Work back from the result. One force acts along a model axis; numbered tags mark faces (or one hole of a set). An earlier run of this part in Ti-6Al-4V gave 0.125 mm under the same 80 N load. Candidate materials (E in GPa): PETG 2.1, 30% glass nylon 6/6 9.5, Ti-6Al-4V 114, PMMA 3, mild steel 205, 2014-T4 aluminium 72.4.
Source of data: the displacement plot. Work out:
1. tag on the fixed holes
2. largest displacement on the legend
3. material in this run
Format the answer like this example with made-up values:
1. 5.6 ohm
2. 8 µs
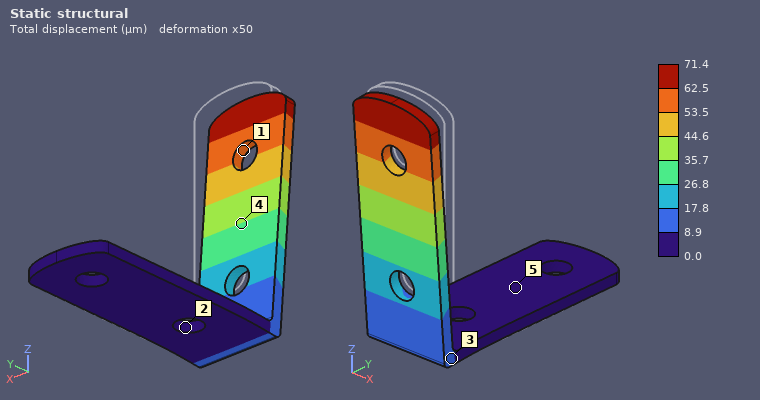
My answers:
1. 2
2. 71.4 µm
3. mild steel
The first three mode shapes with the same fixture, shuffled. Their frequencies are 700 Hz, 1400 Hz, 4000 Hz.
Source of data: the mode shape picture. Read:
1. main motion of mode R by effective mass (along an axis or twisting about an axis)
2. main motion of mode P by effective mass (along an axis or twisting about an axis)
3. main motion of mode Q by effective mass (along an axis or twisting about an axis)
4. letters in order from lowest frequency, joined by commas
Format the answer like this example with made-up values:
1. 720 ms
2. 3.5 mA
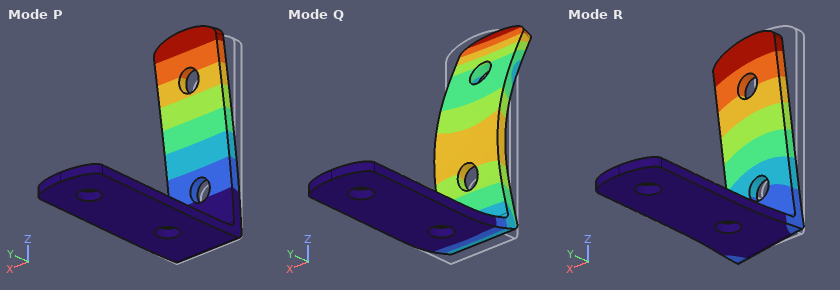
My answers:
1. along X
2. along Y
3. along Z
4. P, R, Q
